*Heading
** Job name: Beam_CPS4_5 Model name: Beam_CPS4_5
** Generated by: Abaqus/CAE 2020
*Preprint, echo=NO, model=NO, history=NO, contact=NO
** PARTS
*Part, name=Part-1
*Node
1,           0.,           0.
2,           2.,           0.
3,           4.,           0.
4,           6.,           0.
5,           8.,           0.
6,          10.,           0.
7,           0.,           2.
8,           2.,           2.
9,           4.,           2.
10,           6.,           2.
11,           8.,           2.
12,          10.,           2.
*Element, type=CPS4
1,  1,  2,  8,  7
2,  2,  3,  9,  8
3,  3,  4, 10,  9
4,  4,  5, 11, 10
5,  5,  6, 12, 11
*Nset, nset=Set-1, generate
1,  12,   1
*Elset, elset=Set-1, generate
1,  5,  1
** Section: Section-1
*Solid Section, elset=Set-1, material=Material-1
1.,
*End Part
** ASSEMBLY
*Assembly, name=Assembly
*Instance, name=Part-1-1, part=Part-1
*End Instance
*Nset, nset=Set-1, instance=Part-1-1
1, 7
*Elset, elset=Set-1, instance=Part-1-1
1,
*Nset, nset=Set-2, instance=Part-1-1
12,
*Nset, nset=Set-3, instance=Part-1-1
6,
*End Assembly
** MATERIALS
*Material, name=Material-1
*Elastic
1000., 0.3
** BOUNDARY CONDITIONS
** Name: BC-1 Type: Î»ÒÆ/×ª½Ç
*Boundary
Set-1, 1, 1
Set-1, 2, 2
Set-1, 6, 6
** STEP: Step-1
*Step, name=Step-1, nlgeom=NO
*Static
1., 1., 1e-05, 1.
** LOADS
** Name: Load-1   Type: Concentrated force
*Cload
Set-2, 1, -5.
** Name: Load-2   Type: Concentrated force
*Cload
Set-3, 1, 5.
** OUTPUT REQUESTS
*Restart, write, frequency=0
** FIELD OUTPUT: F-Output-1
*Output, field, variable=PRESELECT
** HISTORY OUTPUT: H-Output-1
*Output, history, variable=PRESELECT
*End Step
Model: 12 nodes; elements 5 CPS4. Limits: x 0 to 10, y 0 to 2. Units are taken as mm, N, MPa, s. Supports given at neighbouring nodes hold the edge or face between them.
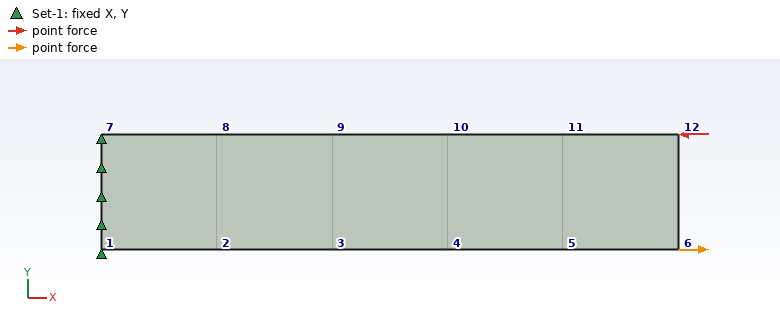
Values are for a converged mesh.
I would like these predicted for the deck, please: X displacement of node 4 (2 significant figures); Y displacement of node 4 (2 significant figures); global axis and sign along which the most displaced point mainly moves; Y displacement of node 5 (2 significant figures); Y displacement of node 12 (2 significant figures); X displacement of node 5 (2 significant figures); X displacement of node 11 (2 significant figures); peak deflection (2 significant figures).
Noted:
0.089 mm
0.27 mm
+Y
0.48 mm
0.75 mm
0.12 mm
-0.12 mm
0.77 mm
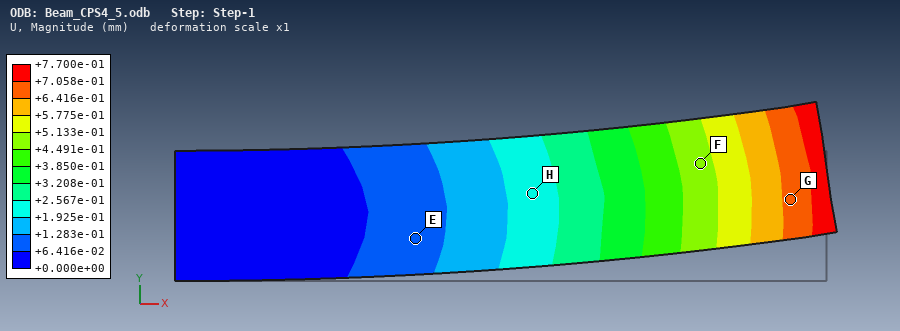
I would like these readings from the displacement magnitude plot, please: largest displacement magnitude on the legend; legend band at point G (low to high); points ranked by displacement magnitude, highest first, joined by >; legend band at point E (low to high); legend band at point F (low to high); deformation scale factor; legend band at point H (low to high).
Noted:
+7.700e-01 mm
+6.416e-01 to +7.058e-01 mm
G > F > H > E
+6.416e-02 to +1.283e-01 mm
+4.491e-01 to +5.133e-01 mm
1
+1.925e-01 to +2.567e-01 mm
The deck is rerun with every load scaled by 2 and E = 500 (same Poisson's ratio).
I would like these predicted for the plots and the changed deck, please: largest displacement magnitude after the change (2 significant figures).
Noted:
3.1 mm
